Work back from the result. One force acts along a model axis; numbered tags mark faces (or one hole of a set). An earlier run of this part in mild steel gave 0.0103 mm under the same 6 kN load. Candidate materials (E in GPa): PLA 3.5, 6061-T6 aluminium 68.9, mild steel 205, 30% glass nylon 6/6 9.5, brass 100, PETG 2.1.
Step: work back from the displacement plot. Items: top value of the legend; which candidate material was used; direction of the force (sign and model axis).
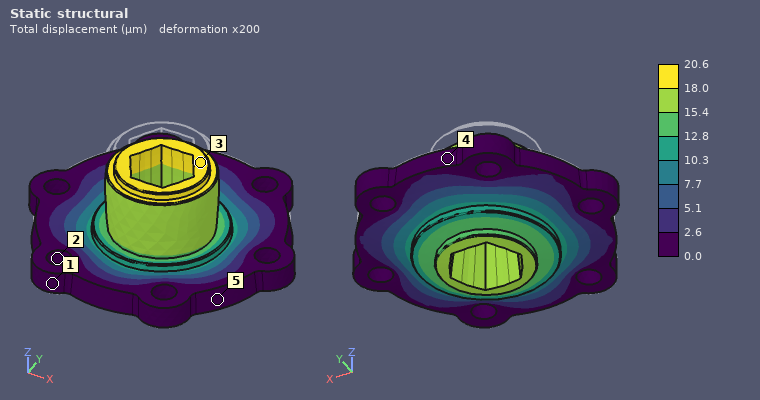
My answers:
20.6 µm
brass
-Z
